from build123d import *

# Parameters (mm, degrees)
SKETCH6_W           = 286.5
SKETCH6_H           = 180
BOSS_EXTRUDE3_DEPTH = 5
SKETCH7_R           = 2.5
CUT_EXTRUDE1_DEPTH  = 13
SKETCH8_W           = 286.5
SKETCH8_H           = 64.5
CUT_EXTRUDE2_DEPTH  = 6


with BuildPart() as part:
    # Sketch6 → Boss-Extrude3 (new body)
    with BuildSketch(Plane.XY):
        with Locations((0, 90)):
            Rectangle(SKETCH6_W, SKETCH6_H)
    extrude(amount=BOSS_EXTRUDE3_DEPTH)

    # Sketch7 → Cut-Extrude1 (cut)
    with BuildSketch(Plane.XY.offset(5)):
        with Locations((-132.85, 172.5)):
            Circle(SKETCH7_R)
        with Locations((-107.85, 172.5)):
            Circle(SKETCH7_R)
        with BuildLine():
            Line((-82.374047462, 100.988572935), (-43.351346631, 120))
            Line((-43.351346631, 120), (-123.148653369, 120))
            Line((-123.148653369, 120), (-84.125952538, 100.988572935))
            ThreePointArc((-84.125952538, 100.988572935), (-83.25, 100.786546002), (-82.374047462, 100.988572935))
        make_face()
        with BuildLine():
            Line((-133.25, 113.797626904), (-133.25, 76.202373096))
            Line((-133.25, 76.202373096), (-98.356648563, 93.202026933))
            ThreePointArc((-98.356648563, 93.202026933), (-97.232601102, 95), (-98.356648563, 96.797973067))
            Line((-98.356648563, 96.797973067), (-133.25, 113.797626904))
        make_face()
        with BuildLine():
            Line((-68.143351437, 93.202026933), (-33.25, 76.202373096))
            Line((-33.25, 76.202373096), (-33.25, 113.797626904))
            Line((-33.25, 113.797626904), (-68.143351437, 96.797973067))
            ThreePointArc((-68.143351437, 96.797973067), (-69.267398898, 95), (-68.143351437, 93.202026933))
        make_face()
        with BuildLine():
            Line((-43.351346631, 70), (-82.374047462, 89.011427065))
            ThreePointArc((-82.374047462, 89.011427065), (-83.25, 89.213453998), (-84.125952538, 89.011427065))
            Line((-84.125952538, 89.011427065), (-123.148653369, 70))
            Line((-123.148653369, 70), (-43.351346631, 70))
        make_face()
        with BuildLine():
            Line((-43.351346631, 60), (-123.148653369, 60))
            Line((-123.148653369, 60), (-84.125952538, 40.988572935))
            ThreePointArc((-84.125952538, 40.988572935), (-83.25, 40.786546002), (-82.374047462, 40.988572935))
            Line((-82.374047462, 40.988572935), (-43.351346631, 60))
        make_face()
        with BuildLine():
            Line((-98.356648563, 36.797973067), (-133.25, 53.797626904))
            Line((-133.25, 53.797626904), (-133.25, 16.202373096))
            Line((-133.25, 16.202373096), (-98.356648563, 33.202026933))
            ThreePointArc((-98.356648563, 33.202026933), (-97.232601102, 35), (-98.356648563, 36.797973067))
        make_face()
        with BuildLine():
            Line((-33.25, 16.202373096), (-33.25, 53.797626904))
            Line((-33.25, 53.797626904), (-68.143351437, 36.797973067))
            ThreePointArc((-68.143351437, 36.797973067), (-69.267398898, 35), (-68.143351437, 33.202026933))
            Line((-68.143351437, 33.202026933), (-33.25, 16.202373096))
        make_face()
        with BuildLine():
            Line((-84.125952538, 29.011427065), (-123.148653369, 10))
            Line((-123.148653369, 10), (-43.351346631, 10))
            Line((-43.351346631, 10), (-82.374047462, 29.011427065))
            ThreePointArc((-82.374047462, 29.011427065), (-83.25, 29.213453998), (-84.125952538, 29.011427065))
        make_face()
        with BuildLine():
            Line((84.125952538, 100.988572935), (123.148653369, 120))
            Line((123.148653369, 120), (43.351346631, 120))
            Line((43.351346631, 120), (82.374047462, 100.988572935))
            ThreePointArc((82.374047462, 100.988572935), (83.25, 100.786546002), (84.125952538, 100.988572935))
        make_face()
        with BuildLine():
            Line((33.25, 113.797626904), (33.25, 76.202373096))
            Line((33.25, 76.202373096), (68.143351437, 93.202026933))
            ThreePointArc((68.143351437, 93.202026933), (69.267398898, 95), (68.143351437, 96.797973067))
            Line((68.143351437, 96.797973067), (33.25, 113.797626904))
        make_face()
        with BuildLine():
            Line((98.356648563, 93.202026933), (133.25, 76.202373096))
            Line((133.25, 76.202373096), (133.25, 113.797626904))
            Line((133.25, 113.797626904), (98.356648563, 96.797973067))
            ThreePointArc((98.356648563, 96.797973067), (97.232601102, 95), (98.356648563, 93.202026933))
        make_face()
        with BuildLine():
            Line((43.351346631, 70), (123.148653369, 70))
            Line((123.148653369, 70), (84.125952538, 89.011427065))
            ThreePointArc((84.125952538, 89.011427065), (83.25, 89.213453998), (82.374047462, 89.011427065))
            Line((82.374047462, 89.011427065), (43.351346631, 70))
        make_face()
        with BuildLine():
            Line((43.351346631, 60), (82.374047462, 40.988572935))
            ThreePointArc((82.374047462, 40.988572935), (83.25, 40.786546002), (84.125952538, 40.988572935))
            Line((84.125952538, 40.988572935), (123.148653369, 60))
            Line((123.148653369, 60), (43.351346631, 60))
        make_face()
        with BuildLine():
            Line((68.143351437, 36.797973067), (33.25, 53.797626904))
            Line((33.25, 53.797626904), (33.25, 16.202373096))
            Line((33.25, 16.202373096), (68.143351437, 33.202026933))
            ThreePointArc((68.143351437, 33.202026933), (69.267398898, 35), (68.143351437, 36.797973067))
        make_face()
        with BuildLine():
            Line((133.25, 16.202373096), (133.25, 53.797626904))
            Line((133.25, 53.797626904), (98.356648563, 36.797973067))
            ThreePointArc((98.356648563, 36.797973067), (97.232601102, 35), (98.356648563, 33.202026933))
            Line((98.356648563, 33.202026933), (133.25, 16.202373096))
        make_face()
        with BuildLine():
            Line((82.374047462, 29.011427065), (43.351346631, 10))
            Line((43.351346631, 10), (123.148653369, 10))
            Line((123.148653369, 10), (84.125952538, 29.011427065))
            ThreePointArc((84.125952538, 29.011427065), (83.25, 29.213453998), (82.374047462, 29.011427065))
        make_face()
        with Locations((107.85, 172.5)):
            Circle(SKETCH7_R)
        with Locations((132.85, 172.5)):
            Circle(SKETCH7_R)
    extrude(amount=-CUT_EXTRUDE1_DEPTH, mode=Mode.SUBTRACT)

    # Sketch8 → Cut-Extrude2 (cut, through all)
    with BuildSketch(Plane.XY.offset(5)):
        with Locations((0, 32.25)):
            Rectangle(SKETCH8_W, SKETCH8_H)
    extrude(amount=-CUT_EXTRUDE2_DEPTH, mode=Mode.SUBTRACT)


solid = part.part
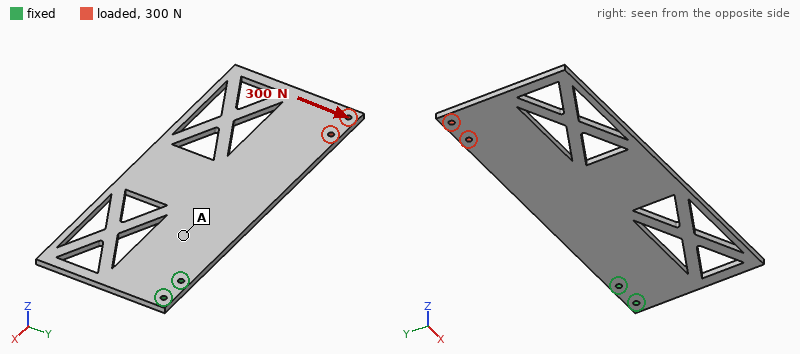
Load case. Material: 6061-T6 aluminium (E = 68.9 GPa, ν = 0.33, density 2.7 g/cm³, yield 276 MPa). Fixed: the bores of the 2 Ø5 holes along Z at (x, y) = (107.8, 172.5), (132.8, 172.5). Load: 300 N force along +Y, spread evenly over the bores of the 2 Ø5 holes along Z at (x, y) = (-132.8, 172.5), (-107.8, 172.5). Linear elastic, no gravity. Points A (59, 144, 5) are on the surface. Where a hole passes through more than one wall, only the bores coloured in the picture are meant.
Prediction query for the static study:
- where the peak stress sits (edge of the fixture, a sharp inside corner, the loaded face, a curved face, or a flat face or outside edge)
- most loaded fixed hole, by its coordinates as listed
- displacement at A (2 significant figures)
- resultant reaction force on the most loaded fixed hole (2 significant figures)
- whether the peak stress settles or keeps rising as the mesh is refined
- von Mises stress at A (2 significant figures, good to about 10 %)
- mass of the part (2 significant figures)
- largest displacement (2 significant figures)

edge of the fixture
(107.8, 172.5)
0.057 mm
2.7 kN
keeps rising
4.5 MPa
360 g
0.32 mm
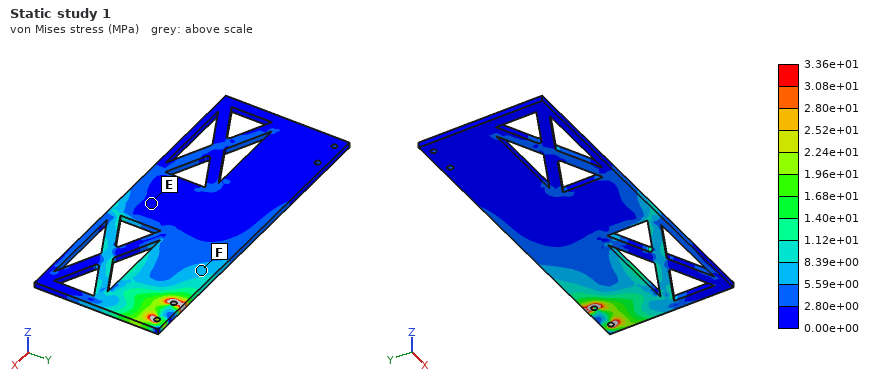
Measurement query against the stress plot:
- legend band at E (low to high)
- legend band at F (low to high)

0.00e+00 to 2.80e+00 MPa
5.59e+00 to 8.39e+00 MPa
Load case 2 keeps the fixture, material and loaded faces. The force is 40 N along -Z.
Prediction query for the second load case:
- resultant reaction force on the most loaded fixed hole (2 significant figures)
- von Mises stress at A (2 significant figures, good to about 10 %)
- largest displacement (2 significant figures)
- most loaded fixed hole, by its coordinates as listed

240 N
21 MPa
3.7 mm
(107.8, 172.5)
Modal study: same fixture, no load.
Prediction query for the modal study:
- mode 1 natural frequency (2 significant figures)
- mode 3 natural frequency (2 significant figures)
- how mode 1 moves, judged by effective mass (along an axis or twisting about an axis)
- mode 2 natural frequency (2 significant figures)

54 Hz
350 Hz
along Z
190 Hz
